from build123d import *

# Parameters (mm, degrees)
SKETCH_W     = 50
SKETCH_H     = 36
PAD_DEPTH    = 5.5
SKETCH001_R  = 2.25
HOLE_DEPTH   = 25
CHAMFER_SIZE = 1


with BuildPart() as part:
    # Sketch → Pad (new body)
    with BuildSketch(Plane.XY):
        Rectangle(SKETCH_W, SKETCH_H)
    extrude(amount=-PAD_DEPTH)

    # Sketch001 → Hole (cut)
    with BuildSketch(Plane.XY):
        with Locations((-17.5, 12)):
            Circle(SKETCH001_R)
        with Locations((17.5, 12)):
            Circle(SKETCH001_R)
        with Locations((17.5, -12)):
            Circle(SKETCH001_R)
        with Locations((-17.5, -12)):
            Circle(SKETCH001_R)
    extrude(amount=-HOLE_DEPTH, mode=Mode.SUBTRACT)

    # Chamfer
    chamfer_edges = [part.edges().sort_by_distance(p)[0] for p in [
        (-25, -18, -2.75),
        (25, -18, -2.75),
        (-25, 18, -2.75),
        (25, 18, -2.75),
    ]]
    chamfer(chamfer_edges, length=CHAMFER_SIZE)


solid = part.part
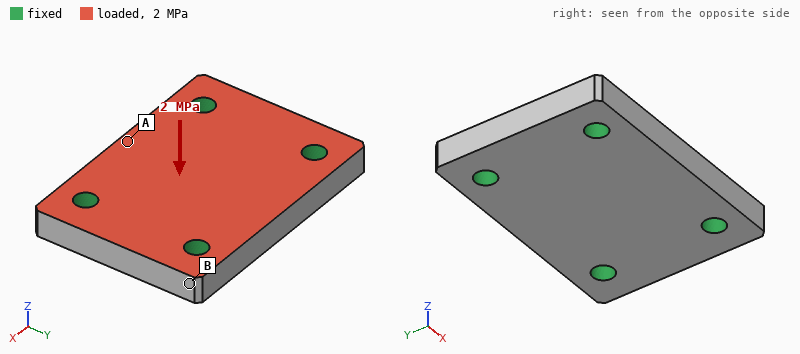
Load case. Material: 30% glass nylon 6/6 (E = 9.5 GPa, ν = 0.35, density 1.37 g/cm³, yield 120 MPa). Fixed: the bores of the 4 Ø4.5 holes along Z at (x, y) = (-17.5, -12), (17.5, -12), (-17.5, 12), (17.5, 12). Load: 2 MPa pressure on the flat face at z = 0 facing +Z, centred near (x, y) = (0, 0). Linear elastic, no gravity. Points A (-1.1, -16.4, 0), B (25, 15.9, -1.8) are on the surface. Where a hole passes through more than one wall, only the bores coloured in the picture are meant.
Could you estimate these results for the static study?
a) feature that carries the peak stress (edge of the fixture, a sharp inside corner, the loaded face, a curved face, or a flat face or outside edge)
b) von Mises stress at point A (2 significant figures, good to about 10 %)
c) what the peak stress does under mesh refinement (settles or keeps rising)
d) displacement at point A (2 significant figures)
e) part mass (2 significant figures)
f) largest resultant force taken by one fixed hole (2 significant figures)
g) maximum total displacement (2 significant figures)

edge of the fixture
19 MPa
keeps rising
70 µm
13 g
870 N
81 µm
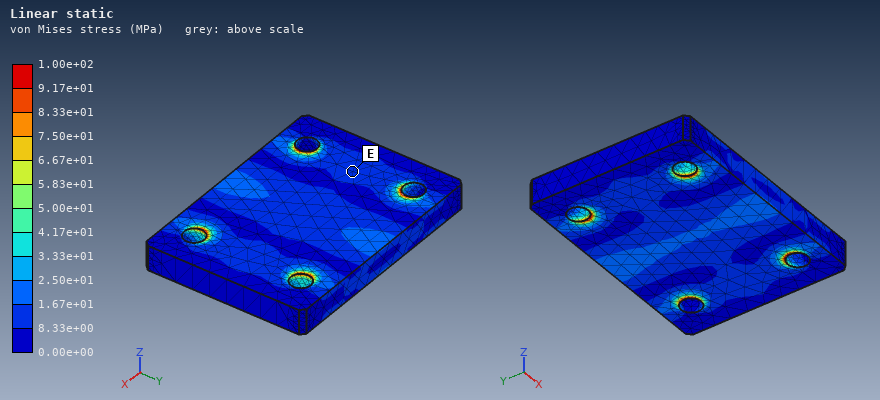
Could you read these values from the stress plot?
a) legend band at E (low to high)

8.33e+00 to 1.67e+01 MPa
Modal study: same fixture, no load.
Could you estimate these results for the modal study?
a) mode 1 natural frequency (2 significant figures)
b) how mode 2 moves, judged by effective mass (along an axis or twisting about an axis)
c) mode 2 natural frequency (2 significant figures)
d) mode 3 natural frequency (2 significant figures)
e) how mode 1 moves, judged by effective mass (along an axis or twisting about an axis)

10 kHz
twisting about X
13 kHz
18 kHz
along Z
